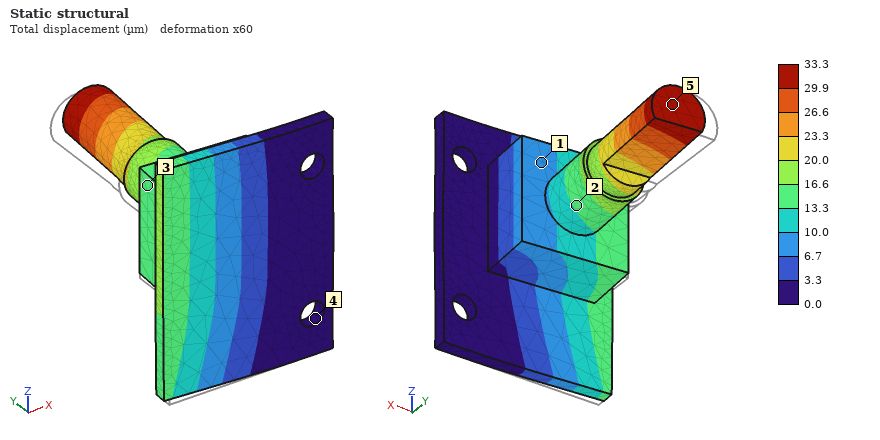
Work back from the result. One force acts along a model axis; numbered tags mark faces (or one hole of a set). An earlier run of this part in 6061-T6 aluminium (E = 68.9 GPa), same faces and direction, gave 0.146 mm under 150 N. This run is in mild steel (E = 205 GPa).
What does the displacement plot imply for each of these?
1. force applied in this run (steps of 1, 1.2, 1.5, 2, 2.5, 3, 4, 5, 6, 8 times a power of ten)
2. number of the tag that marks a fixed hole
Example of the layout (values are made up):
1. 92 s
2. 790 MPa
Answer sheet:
1. 100 N
2. 4
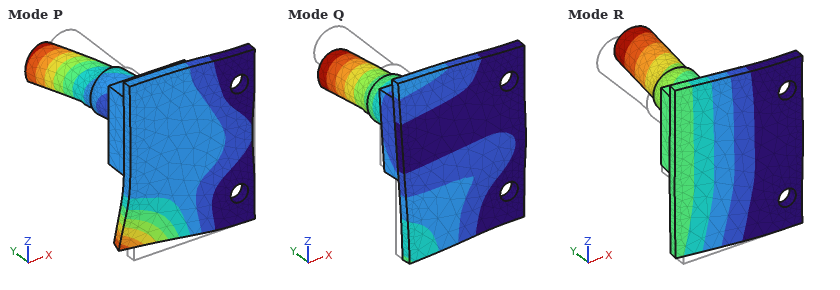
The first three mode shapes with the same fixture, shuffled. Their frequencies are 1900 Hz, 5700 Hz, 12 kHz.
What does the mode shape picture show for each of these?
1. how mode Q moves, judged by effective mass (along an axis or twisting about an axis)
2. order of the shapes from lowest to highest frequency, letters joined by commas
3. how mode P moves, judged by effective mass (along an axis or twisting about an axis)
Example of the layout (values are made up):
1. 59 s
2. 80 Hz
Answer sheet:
1. along Z
2. R, Q, P
3. along Y
